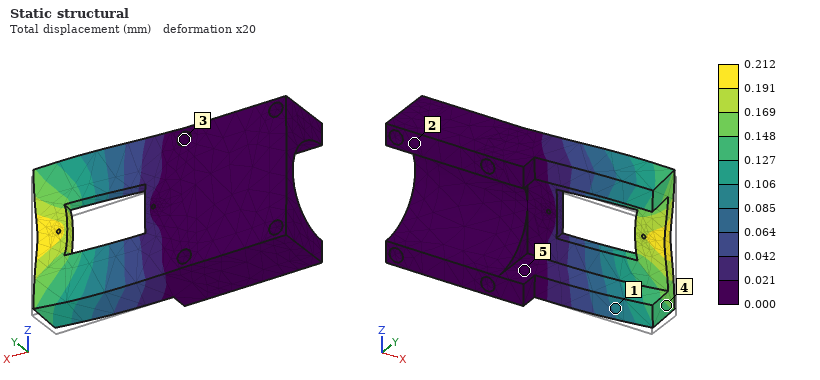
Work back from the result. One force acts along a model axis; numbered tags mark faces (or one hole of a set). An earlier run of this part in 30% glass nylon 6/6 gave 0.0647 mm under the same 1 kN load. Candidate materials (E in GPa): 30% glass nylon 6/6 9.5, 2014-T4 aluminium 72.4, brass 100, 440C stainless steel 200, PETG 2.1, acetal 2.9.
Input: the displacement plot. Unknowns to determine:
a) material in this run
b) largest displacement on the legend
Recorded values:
acetal
0.212 mm
